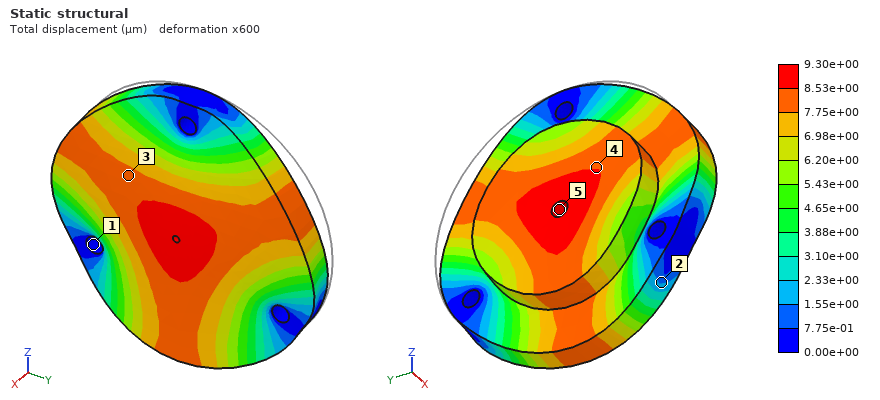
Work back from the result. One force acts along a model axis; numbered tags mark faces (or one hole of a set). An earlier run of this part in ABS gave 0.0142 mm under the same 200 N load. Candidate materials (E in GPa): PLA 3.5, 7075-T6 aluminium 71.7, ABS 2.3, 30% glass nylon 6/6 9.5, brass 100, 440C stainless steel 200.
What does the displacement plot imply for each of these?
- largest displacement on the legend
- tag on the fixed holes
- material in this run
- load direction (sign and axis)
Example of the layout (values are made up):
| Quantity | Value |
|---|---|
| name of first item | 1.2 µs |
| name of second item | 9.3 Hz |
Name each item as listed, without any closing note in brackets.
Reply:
| Quantity | Value |
|---|---|
| largest displacement on the legend | 9.30e+00 µm |
| tag on the fixed holes | 1 |
| material in this run | PLA |
| load direction | +X |
